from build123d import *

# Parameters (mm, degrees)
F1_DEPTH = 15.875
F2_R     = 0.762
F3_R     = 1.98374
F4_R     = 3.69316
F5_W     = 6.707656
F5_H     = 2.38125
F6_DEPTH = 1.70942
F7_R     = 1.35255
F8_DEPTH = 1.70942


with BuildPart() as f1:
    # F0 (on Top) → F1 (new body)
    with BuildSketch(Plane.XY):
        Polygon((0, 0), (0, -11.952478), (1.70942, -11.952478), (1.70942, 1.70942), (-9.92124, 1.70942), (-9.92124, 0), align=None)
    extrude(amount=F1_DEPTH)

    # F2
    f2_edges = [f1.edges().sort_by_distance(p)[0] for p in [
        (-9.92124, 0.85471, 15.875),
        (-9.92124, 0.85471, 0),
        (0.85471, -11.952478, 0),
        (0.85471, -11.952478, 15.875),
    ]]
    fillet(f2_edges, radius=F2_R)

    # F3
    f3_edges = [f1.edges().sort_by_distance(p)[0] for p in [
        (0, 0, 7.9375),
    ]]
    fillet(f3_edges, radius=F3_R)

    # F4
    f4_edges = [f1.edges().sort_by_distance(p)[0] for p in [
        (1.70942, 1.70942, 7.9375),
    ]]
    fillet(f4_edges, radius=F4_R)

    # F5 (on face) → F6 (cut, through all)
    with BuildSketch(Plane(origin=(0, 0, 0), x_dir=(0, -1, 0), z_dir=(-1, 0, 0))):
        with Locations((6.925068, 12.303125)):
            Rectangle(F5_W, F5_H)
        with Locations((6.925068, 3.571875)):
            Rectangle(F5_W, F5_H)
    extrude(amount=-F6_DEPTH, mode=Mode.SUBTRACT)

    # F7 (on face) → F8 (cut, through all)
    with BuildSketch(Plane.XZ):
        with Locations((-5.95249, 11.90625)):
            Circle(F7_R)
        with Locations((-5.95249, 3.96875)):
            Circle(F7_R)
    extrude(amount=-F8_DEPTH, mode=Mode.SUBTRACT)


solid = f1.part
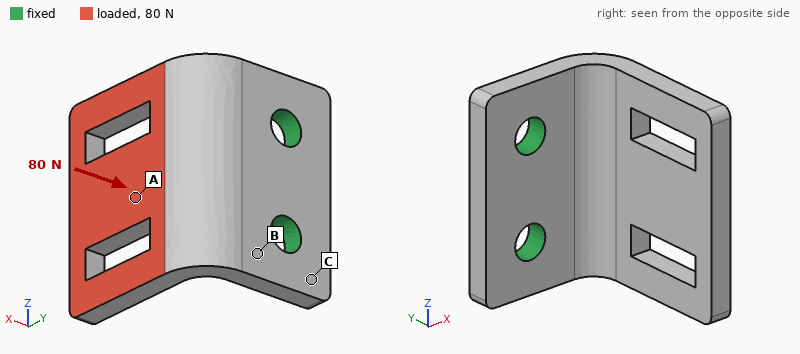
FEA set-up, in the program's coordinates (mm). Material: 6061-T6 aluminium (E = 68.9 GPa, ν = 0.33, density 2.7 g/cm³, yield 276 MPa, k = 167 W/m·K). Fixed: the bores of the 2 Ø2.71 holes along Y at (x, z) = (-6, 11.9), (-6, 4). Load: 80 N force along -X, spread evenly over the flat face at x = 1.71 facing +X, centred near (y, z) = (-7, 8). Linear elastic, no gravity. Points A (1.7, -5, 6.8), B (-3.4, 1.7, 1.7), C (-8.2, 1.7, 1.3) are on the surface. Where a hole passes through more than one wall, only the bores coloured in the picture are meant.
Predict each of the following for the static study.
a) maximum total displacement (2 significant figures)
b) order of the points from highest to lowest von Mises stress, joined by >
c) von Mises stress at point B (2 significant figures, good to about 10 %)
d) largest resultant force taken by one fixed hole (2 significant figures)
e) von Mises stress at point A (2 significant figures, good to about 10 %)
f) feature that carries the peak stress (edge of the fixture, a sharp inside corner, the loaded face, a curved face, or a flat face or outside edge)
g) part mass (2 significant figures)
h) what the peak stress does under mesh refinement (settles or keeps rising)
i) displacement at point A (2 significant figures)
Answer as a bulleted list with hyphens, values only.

- 0.15 mm
- B > A > C
- 68 MPa
- 41 N
- 34 MPa
- edge of the fixture
- 1.4 g
- keeps rising
- 0.064 mm
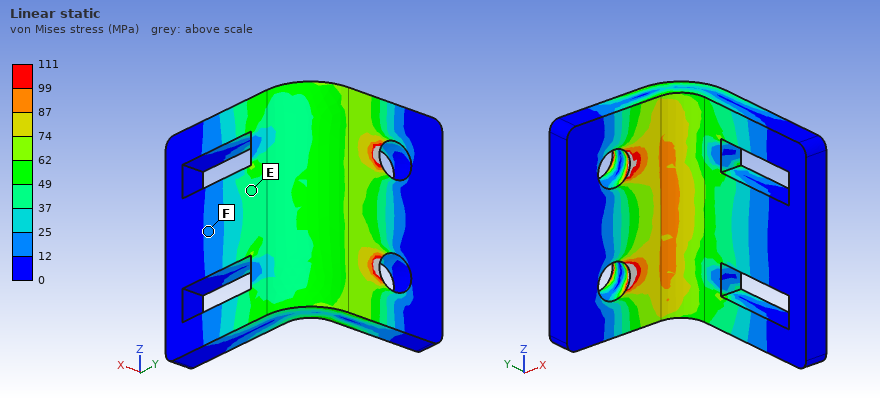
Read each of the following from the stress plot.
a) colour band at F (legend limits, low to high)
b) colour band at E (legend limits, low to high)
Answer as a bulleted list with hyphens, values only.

- 12 to 25 MPa
- 37 to 49 MPa
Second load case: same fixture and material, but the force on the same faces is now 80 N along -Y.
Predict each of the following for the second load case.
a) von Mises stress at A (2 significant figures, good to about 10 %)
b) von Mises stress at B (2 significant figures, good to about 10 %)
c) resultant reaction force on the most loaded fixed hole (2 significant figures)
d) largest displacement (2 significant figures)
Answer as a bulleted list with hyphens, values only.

- 10 MPa
- 44 MPa
- 40 N
- 64 µm
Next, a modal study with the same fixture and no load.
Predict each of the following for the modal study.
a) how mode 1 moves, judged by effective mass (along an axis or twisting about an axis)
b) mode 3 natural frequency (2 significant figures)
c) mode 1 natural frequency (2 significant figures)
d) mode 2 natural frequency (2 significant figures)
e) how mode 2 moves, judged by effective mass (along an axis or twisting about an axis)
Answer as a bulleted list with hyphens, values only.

- along X
- 17 kHz
- 5700 Hz
- 10 kHz
- along Z
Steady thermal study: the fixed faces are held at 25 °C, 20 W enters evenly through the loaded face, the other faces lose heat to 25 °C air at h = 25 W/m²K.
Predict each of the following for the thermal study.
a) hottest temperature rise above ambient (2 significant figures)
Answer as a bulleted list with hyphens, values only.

- 64 K
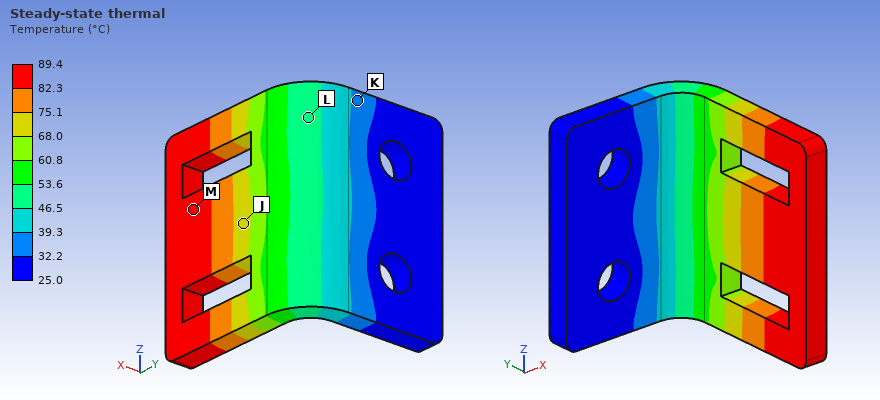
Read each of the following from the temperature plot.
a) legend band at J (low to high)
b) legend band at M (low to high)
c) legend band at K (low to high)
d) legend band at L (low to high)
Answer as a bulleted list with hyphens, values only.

- 68.0 to 75.1 °C
- 82.3 to 89.4 °C
- 32.2 to 39.3 °C
- 46.5 to 53.6 °C
